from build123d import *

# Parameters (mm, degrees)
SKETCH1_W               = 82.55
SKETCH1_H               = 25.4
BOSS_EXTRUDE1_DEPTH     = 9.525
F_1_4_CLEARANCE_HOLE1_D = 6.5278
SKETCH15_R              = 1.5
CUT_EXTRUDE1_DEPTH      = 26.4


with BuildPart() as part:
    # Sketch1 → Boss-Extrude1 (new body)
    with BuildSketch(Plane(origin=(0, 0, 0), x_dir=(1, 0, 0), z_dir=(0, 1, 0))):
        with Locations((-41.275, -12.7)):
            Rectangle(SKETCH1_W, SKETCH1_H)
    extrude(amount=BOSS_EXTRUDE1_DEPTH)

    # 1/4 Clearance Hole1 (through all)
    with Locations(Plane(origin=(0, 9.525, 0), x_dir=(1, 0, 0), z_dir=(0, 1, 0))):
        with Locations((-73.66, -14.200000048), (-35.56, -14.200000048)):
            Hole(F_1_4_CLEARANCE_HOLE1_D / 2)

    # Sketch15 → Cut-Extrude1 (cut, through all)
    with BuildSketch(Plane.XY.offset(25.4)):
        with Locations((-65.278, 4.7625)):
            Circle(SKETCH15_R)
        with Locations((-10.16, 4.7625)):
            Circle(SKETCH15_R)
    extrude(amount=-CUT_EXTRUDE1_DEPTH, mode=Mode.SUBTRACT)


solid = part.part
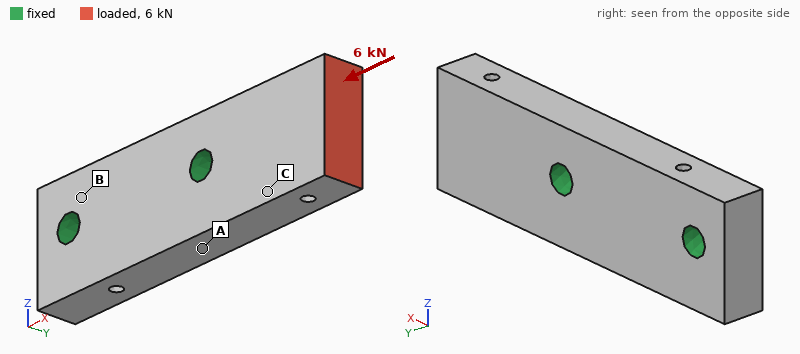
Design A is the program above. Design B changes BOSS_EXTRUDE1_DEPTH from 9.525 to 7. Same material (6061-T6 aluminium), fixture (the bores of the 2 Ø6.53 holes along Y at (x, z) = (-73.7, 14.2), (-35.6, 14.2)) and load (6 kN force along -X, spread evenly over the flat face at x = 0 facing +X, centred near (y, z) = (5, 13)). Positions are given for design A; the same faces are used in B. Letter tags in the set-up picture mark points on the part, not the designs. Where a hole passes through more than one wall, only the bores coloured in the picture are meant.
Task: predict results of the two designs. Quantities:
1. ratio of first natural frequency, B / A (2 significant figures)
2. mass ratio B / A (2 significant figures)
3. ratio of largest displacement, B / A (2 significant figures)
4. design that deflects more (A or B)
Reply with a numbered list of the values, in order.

1. 0.77
2. 0.73
3. 1.6
4. B
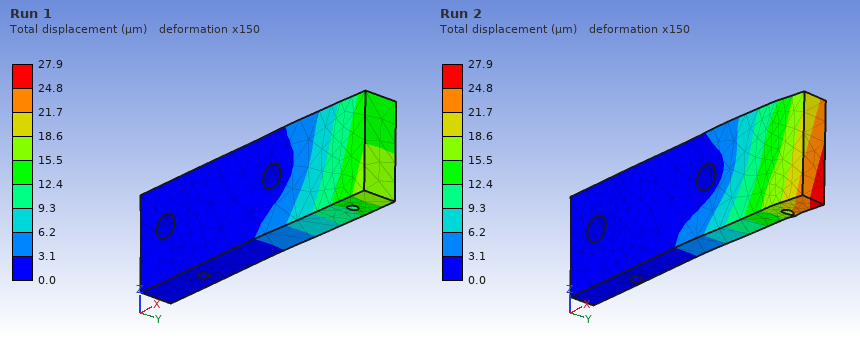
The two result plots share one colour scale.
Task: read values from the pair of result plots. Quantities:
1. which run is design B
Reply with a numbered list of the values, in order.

1. Run 2
